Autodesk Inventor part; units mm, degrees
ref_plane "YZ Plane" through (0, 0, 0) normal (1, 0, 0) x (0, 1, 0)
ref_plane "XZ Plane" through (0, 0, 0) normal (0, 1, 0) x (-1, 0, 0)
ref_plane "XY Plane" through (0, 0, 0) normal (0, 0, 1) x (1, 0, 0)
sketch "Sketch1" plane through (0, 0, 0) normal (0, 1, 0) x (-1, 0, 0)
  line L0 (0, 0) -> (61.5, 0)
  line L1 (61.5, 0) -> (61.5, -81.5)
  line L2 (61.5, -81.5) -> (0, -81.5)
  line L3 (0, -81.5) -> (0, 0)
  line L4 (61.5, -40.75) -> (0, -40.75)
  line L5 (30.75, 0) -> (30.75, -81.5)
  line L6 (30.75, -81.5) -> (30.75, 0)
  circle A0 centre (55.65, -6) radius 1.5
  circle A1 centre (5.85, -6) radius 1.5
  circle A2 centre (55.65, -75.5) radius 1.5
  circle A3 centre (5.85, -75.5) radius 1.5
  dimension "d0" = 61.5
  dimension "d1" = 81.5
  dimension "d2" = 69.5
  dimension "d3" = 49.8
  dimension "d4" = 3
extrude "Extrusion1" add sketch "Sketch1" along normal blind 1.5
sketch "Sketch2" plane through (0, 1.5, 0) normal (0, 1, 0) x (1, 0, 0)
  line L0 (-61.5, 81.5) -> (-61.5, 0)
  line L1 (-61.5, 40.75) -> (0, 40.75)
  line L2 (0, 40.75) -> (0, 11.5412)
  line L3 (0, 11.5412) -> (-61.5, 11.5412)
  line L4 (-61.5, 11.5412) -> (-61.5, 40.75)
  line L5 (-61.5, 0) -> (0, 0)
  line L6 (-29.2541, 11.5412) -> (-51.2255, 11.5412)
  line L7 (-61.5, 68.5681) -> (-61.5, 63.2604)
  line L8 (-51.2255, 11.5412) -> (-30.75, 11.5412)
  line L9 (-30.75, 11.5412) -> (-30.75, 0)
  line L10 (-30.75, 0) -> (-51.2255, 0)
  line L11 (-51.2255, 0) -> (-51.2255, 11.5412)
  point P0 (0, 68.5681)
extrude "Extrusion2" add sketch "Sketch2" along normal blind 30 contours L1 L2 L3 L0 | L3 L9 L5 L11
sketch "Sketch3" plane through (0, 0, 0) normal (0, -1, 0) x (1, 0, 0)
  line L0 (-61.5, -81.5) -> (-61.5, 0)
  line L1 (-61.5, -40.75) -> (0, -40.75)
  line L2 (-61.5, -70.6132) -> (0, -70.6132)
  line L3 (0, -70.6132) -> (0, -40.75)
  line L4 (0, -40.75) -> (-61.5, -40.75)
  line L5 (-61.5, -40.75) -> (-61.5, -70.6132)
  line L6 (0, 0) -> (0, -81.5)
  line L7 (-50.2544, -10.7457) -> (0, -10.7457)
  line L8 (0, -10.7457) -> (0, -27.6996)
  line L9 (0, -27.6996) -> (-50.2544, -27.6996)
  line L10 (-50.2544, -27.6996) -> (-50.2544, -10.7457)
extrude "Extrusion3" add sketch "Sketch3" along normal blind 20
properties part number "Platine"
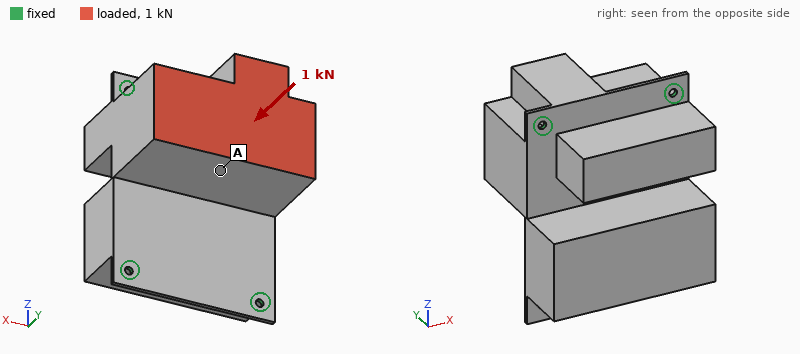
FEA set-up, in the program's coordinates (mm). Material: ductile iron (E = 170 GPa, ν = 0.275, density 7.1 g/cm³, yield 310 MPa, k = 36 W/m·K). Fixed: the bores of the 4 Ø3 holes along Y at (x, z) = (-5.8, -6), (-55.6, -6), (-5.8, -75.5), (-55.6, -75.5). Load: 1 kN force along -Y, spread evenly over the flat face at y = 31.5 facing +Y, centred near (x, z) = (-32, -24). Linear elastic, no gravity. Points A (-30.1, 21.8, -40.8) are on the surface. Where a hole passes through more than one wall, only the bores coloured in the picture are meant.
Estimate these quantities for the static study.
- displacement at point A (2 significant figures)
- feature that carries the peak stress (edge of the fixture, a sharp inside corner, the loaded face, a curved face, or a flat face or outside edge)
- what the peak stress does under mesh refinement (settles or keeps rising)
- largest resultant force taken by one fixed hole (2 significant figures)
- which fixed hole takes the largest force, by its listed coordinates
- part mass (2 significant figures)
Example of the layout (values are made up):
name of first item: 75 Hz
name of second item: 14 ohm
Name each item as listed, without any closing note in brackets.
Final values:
displacement at point A: 46 µm
feature that carries the peak stress: edge of the fixture
what the peak stress does under mesh refinement: keeps rising
largest resultant force taken by one fixed hole: 420 N
which fixed hole takes the largest force, by its listed coordinates: (-55.6, -6)
part mass: 870 g
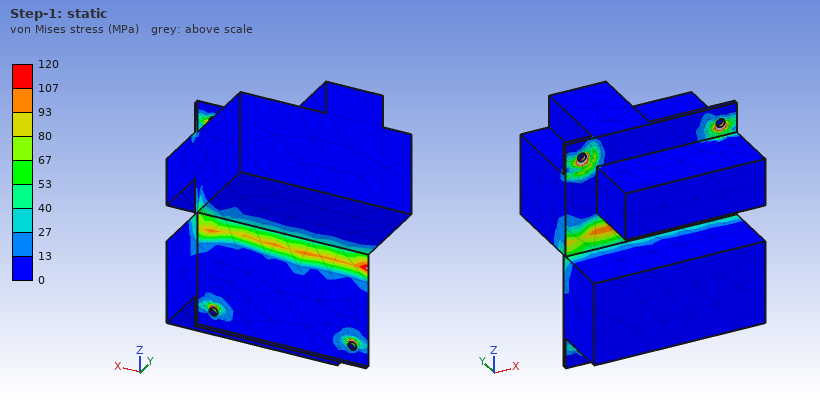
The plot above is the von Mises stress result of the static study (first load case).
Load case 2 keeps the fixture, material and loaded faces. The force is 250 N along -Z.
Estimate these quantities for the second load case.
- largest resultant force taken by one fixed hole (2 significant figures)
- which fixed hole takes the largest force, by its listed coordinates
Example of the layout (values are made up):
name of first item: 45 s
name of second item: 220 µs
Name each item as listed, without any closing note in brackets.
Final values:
largest resultant force taken by one fixed hole: 120 N
which fixed hole takes the largest force, by its listed coordinates: (-55.6, -6)
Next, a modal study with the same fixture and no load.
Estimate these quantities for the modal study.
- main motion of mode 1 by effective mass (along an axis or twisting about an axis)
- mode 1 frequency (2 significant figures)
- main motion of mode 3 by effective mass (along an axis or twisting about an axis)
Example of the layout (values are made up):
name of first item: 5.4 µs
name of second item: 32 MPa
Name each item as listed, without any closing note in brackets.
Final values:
main motion of mode 1 by effective mass: along Y
mode 1 frequency: 850 Hz
main motion of mode 3 by effective mass: along Y
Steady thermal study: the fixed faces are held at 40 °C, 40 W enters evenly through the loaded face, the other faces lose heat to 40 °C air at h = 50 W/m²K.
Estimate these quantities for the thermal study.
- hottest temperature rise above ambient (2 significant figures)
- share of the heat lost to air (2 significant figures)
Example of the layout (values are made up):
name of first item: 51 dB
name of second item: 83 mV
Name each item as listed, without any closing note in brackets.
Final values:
hottest temperature rise above ambient: 48 K
share of the heat lost to air: 70 %
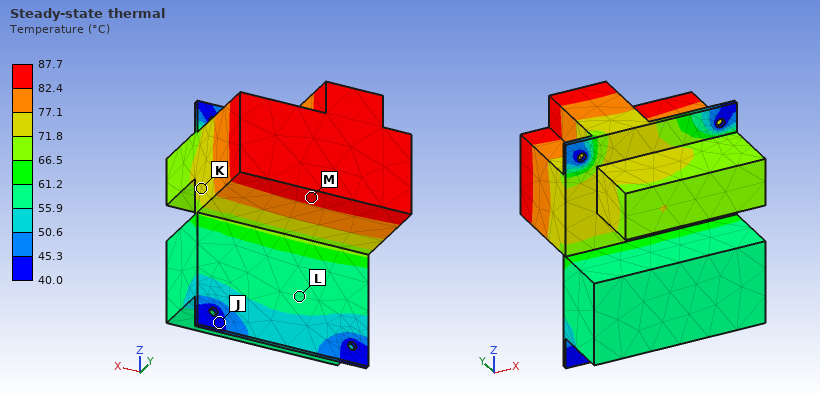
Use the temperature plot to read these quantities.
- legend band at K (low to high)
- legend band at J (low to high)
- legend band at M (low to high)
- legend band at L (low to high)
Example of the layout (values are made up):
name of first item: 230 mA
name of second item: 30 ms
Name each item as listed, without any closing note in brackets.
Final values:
legend band at K: 71.8 to 77.1 °C
legend band at J: 40.0 to 45.3 °C
legend band at M: 82.4 to 87.7 °C
legend band at L: 55.9 to 61.2 °C
